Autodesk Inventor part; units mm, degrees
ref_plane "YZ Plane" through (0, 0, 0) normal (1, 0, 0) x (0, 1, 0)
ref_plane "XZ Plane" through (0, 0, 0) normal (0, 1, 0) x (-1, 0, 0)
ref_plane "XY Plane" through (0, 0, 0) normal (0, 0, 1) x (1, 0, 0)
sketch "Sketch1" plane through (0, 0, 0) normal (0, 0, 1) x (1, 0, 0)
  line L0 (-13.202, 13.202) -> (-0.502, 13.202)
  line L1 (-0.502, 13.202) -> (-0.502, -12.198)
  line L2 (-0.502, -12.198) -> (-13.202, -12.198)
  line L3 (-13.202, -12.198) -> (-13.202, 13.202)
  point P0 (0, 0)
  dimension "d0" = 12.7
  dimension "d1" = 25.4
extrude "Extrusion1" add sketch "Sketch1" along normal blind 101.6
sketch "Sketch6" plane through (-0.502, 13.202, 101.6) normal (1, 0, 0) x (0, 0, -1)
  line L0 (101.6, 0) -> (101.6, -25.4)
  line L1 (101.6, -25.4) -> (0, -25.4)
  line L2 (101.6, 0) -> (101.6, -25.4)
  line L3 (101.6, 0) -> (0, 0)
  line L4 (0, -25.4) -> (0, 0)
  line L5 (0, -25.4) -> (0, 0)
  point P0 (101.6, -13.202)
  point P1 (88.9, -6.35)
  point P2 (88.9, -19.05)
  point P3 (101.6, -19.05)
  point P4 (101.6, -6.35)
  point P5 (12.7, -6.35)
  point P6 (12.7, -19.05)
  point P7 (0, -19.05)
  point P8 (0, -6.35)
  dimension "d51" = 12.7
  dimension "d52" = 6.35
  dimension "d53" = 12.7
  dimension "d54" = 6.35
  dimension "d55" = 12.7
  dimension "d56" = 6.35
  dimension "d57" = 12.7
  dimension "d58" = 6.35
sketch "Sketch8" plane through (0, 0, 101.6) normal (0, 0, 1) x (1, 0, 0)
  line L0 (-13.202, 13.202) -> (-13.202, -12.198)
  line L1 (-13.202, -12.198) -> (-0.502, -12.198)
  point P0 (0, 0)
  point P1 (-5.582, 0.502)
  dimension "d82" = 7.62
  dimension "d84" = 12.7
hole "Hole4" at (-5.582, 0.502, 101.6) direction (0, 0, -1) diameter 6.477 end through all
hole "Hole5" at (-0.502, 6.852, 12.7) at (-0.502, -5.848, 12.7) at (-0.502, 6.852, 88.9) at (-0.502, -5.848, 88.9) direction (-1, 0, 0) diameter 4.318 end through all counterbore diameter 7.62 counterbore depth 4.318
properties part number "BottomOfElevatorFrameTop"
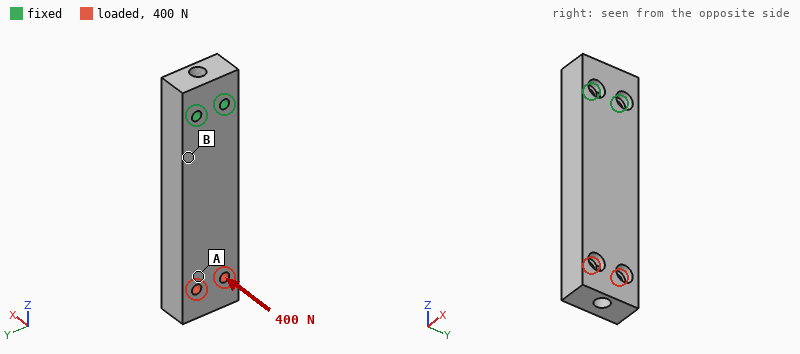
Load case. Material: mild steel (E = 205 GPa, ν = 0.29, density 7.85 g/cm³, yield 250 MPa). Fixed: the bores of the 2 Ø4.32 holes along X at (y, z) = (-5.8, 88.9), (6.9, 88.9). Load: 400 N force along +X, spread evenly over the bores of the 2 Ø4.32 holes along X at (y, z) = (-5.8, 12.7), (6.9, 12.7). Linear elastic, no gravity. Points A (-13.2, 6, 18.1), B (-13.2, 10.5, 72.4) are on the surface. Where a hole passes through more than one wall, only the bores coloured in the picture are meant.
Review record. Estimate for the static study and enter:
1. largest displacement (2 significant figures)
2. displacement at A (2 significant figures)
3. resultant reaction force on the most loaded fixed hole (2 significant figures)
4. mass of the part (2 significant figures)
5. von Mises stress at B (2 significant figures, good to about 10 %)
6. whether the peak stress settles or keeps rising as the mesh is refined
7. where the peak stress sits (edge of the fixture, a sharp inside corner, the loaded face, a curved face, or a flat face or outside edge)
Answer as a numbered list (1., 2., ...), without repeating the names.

1. 0.11 mm
2. 0.083 mm
3. 220 N
4. 220 g
5. 35 MPa
6. keeps rising
7. edge of the fixture
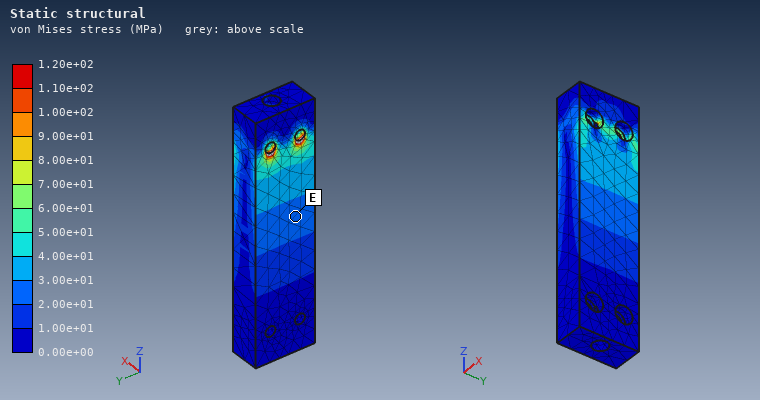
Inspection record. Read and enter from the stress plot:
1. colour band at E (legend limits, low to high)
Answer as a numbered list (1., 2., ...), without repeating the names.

1. 2.00e+01 to 3.00e+01 MPa
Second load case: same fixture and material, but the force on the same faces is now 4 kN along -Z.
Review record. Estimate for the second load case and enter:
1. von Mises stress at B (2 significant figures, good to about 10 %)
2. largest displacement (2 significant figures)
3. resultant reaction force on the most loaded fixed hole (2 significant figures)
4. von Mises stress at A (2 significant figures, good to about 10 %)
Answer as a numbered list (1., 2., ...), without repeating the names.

1. 25 MPa
2. 33 µm
3. 2.0 kN
4. 24 MPa
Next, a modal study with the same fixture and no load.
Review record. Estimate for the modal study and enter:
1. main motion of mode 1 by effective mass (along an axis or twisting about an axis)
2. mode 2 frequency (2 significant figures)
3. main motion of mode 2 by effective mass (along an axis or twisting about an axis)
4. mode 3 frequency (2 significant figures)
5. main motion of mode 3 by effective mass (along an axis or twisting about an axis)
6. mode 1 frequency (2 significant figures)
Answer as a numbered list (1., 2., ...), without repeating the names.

1. along X
2. 2400 Hz
3. along Y
4. 6500 Hz
5. twisting about Z
6. 1200 Hz
